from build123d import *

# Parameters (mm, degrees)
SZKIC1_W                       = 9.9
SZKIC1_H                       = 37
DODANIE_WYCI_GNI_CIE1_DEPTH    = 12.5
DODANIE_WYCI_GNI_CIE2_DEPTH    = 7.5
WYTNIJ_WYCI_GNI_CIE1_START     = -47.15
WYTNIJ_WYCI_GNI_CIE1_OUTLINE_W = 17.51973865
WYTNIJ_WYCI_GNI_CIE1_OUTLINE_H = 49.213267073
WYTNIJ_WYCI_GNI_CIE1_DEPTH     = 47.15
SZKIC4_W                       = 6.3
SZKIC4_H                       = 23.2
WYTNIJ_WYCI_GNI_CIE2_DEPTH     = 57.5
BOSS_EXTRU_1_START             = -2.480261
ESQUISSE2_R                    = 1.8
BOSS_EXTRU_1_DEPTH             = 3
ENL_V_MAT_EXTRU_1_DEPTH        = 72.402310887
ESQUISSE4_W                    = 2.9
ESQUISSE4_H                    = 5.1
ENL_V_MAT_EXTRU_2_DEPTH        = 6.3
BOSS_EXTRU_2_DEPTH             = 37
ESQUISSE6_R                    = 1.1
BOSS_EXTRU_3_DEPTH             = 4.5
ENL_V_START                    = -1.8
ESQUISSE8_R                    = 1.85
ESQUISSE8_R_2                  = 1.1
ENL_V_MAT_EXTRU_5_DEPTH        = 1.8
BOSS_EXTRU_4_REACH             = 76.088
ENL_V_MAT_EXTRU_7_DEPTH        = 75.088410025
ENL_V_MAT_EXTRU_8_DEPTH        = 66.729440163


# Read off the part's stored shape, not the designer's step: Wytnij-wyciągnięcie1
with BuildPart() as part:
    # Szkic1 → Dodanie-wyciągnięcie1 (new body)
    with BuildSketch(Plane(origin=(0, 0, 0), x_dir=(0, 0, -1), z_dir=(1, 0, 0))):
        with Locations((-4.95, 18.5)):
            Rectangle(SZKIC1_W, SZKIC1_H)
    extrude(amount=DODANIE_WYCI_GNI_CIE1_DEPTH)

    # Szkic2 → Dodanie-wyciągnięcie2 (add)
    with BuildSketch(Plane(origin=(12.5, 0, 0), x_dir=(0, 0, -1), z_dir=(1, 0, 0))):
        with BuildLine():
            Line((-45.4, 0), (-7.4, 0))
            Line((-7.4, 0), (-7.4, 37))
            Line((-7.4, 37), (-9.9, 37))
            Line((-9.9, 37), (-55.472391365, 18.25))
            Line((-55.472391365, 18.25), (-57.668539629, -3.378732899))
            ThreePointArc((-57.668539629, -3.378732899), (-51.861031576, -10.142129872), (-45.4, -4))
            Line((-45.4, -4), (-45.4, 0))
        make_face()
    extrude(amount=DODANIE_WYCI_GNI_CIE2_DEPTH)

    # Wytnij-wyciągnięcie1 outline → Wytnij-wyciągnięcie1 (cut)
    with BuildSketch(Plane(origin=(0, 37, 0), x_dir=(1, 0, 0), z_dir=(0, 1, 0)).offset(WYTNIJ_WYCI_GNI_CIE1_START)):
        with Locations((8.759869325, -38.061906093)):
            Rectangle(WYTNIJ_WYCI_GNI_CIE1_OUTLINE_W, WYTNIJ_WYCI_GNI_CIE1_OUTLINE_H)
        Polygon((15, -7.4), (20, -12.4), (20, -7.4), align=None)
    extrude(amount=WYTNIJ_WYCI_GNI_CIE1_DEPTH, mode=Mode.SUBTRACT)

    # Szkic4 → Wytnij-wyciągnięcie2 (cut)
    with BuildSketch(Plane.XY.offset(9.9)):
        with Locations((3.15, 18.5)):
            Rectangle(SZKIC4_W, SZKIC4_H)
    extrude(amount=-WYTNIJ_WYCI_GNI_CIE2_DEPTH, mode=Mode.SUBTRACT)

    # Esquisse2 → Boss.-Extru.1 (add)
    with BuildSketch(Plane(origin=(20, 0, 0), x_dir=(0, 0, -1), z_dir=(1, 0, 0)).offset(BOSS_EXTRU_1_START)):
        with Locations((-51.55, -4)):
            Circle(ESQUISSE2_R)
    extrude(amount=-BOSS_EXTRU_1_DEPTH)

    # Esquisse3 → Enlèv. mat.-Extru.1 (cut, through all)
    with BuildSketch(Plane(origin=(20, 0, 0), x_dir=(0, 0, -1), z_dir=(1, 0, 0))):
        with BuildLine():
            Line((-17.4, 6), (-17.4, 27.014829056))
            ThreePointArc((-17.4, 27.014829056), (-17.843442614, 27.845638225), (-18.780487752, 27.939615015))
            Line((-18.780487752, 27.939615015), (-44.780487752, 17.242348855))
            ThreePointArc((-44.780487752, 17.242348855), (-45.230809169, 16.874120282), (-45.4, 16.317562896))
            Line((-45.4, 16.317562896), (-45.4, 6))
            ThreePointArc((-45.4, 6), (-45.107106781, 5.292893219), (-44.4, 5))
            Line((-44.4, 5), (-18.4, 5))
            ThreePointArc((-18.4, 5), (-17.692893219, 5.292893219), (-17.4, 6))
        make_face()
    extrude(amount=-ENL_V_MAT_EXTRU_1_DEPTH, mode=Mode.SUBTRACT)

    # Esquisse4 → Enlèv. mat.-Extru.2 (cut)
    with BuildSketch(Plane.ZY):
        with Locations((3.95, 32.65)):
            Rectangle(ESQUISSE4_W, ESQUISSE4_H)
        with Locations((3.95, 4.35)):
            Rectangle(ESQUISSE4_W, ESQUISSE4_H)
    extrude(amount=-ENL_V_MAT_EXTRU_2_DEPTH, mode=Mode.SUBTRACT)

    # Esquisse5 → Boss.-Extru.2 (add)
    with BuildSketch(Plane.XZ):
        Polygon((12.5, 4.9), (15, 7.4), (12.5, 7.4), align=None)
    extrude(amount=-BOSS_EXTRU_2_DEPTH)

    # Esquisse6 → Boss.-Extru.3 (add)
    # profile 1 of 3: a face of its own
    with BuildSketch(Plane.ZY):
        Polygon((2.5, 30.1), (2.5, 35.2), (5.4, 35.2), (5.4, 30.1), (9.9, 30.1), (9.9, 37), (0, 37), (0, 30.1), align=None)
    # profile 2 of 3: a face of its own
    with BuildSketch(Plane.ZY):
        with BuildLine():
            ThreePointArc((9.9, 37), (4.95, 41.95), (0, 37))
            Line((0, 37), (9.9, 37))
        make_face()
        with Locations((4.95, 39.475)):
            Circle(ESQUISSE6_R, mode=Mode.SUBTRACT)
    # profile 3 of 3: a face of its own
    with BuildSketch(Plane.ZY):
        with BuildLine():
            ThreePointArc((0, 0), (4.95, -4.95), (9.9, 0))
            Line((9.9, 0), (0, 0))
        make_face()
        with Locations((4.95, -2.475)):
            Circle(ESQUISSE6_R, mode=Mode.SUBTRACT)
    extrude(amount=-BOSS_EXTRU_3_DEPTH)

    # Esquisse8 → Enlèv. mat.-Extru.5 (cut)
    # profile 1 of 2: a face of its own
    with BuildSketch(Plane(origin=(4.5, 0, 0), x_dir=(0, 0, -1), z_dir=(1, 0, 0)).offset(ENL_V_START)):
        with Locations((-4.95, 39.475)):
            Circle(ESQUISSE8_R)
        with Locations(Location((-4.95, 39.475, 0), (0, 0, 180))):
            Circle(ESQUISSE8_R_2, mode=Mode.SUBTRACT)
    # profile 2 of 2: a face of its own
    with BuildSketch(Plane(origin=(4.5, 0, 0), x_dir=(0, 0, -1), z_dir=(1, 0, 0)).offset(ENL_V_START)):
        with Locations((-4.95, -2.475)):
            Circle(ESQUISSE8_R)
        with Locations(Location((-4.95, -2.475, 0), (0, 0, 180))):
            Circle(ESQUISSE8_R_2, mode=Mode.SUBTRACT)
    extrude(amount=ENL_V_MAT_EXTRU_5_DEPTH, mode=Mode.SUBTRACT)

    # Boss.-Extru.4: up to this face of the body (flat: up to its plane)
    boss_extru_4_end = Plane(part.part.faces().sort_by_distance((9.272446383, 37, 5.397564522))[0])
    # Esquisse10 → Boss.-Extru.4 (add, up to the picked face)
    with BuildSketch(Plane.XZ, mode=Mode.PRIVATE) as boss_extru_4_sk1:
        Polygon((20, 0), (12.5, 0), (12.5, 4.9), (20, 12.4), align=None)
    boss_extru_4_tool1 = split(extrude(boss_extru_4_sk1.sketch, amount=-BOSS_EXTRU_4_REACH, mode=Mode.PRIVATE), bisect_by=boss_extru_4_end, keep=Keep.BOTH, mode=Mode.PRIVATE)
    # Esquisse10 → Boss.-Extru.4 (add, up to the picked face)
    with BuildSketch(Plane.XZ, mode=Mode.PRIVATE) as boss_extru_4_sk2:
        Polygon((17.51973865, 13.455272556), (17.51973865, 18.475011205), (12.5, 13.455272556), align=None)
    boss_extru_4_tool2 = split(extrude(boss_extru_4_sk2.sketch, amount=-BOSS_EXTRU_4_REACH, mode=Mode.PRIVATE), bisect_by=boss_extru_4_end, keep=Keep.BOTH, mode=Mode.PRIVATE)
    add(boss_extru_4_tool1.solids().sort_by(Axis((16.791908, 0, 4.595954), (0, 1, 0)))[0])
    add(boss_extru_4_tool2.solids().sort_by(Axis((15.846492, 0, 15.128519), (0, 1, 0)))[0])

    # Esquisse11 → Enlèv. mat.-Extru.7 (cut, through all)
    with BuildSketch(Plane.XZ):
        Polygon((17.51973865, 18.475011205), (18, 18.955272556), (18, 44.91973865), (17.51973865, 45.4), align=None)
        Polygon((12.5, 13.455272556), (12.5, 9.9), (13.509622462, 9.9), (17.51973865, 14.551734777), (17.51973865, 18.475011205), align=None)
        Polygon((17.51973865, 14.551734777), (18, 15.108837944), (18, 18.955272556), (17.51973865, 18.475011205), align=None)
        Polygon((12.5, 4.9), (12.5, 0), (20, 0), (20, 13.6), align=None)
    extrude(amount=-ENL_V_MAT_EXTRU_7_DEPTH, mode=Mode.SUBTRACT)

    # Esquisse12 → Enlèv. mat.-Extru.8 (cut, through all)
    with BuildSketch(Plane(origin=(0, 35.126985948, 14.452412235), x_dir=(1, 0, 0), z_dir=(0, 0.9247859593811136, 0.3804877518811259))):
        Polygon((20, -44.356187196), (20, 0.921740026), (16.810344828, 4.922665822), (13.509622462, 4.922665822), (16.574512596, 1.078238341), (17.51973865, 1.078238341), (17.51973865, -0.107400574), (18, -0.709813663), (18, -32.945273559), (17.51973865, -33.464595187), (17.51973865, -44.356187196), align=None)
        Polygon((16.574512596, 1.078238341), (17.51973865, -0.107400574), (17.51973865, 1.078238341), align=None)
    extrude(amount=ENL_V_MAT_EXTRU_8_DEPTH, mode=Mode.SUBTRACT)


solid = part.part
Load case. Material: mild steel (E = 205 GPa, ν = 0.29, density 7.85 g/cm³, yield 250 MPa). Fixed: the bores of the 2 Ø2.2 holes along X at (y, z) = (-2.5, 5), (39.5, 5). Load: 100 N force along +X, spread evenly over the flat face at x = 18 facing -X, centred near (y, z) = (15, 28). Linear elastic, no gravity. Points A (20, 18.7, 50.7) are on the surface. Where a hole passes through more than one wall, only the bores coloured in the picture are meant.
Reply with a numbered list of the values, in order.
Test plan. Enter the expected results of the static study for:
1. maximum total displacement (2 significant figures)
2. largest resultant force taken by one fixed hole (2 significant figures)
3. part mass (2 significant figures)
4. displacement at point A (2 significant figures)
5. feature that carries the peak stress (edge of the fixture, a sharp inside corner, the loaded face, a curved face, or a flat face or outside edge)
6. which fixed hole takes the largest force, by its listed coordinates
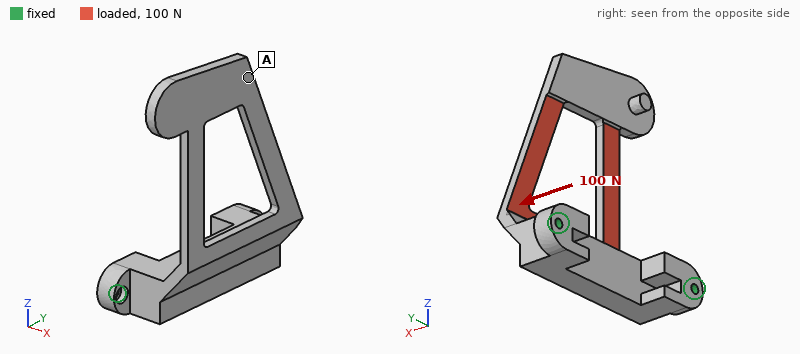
1. 0.46 mm
2. 74 N
3. 46 g
4. 0.36 mm
5. a curved face
6. (-2.5, 5)
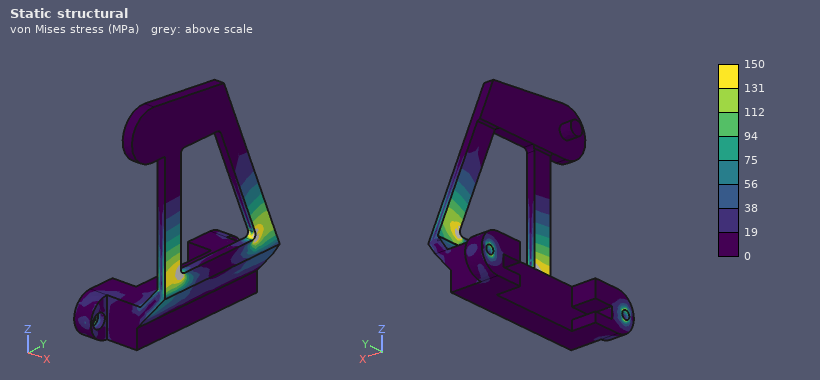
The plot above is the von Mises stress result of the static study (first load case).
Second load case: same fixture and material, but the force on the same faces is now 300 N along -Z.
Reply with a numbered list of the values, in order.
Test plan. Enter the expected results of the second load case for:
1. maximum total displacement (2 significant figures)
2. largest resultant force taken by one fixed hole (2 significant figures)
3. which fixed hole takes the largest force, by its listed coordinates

1. 47 µm
2. 170 N
3. (-2.5, 5)
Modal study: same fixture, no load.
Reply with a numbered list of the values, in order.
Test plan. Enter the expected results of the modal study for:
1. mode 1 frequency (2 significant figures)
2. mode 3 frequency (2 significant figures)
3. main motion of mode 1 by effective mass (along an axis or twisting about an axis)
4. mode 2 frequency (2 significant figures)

1. 480 Hz
2. 2600 Hz
3. along X
4. 1800 Hz
